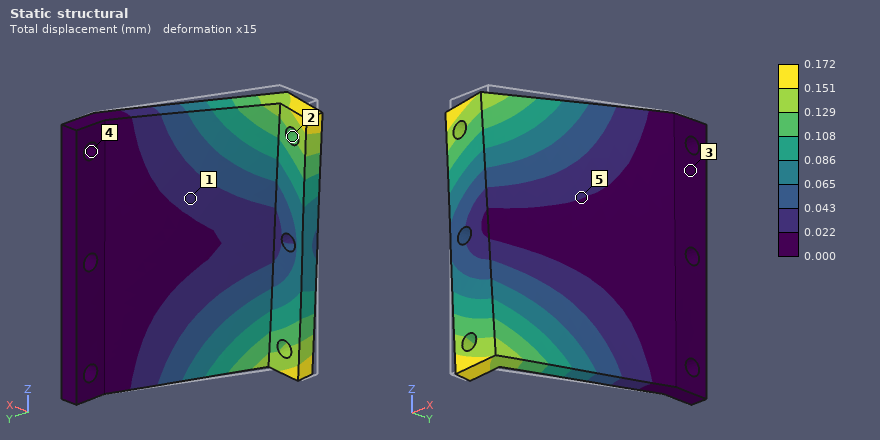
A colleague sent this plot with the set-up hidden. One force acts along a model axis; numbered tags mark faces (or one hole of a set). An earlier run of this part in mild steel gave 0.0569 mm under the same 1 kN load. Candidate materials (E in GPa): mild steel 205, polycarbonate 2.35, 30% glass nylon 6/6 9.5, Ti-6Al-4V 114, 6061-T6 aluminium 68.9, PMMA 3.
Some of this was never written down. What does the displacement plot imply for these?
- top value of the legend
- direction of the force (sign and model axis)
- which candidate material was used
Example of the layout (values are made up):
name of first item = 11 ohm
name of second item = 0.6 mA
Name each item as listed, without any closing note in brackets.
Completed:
top value of the legend = 0.172 mm
direction of the force = -Z
which candidate material was used = 6061-T6 aluminium
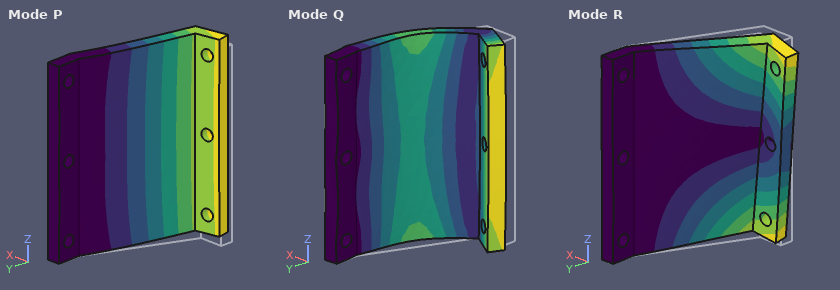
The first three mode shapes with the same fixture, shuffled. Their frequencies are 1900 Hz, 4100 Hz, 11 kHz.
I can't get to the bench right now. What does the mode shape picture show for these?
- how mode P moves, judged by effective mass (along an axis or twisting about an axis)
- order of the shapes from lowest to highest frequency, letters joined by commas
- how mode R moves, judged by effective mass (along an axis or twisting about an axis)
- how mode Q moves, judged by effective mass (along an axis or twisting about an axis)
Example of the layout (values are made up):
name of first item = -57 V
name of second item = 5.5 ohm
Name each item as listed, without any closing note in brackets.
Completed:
how mode P moves, judged by effective mass = along X
order of the shapes from lowest to highest frequency, letters joined by commas = P, R, Q
how mode R moves, judged by effective mass = twisting about Y
how mode Q moves, judged by effective mass = along X
